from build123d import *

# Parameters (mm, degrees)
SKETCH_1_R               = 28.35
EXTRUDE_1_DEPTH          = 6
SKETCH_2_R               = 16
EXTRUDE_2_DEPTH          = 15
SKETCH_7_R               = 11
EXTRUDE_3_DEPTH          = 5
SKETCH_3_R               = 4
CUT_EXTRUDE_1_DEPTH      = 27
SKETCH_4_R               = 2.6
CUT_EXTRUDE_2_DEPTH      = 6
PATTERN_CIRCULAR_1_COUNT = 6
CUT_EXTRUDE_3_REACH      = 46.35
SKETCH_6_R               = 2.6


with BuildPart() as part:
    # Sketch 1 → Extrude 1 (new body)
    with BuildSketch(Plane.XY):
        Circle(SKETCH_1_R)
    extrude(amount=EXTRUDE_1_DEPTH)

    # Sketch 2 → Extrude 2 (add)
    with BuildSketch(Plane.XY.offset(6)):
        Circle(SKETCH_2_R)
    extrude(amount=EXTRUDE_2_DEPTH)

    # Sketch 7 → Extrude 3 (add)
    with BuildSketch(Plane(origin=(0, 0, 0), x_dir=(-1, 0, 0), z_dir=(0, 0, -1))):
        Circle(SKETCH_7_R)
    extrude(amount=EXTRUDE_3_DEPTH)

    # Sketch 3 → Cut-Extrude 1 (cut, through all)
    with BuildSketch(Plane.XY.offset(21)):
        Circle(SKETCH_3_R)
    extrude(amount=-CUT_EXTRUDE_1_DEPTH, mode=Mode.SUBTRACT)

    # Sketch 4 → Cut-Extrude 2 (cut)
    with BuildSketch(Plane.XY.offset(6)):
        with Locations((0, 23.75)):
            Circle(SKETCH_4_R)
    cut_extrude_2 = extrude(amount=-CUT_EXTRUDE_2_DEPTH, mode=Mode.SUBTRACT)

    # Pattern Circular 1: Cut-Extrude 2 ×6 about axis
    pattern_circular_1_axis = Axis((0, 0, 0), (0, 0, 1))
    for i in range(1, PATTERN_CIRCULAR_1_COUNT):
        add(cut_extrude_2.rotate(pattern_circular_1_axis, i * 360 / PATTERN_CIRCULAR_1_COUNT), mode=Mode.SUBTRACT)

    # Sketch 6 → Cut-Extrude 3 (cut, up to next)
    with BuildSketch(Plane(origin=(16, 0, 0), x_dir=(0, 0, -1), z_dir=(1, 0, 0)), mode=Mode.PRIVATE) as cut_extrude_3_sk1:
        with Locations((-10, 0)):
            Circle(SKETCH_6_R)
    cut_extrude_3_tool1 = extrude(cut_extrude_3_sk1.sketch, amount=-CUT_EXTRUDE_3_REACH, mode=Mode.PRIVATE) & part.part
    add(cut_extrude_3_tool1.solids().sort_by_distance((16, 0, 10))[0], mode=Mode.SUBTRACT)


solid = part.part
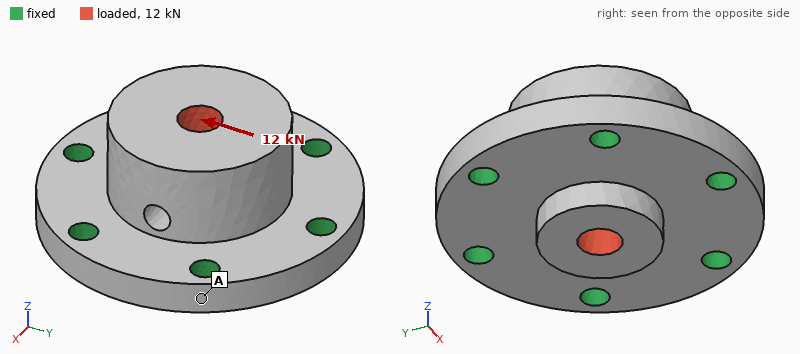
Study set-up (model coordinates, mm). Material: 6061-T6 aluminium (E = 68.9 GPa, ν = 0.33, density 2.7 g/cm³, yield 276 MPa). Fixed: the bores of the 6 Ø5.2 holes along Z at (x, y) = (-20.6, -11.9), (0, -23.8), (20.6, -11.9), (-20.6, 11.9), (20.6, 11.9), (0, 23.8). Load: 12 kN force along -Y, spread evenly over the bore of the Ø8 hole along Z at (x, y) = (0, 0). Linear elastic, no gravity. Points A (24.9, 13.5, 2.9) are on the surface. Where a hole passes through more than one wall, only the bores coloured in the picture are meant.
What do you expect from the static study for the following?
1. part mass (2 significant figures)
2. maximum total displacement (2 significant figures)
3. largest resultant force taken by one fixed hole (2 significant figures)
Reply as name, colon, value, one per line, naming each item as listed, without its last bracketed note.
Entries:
part mass: 72 g
maximum total displacement: 17 µm
largest resultant force taken by one fixed hole: 3.2 kN
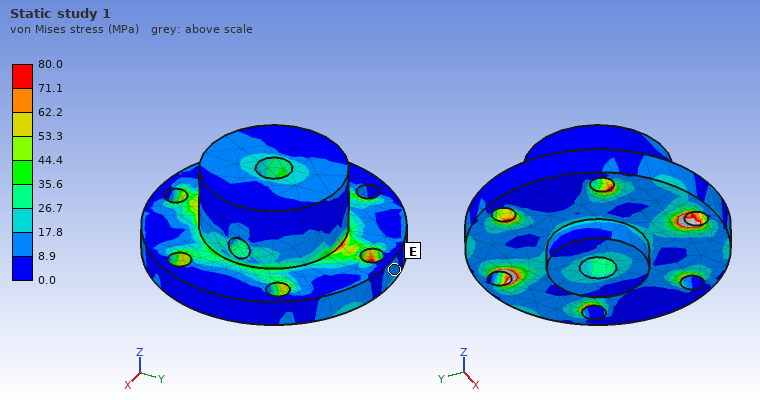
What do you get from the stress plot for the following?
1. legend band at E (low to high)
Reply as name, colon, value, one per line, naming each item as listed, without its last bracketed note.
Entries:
legend band at E: 8.9 to 17.8 MPa
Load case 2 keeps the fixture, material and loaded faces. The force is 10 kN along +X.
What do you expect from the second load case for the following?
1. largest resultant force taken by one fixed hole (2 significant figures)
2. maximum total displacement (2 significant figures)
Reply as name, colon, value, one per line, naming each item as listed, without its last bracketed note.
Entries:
largest resultant force taken by one fixed hole: 2.4 kN
maximum total displacement: 14 µm
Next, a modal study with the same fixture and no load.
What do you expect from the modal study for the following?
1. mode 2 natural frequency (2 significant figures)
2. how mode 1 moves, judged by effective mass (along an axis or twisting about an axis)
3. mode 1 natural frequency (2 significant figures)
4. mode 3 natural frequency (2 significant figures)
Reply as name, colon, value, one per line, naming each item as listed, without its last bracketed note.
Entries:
mode 2 natural frequency: 20 kHz
how mode 1 moves, judged by effective mass: along Z
mode 1 natural frequency: 19 kHz
mode 3 natural frequency: 20 kHz
